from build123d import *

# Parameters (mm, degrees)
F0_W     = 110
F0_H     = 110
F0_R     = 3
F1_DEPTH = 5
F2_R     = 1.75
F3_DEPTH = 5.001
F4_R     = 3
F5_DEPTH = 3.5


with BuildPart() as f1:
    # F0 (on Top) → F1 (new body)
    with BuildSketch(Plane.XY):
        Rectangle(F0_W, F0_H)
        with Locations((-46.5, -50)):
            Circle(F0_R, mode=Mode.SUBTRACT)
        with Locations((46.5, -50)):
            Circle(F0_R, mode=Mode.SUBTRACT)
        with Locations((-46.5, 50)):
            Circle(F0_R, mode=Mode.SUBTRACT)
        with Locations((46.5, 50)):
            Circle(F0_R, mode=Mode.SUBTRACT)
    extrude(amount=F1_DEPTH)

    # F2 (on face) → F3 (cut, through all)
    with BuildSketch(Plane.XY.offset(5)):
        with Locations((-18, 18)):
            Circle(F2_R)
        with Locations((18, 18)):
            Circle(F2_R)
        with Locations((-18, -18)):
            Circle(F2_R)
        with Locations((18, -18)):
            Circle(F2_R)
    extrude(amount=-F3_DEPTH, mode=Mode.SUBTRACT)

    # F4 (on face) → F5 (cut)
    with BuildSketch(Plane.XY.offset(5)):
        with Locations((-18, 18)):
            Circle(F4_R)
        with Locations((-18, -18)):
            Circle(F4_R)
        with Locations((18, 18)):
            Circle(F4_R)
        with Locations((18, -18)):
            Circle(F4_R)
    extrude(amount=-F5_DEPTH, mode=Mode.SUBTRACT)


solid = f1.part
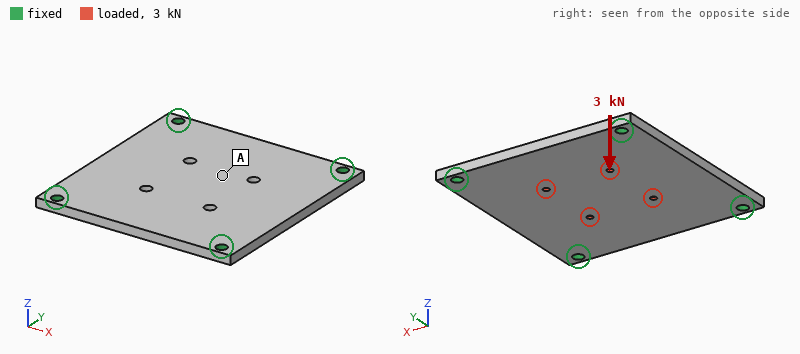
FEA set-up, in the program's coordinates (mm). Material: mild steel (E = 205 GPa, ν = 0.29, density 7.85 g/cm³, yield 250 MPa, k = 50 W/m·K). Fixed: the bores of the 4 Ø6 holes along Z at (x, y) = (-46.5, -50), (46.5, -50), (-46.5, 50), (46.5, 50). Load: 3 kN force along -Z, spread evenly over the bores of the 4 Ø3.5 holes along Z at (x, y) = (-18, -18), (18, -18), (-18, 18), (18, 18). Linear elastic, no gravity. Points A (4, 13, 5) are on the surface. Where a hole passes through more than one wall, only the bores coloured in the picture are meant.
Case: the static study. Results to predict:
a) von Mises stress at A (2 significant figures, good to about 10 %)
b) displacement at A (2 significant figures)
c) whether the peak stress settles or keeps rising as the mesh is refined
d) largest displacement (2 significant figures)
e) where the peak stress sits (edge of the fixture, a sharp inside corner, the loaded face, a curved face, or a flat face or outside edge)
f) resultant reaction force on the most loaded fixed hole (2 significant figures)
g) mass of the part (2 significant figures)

58 MPa
0.12 mm
keeps rising
0.13 mm
edge of the fixture
750 N
470 g
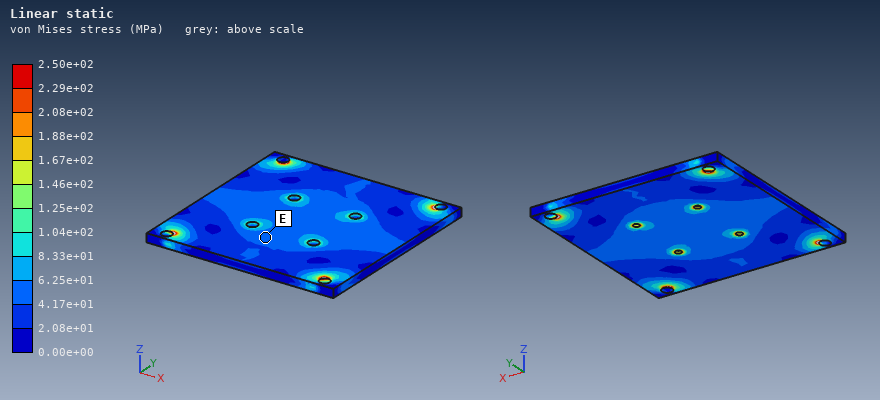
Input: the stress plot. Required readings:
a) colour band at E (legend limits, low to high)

4.17e+01 to 6.25e+01 MPa
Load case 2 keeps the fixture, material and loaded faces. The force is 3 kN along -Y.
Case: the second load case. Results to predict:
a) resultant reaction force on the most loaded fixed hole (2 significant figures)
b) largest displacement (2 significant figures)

830 N
2.9 µm
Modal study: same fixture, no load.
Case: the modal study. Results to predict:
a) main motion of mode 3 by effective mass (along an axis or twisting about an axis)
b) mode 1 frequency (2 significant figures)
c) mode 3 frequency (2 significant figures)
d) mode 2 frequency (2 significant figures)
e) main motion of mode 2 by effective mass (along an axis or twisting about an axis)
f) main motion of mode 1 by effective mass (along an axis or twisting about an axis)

twisting about X
1800 Hz
3300 Hz
3000 Hz
twisting about Y
along Z
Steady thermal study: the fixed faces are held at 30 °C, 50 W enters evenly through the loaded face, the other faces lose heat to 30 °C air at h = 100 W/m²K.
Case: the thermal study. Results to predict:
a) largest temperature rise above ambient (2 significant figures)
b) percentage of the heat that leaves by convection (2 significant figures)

52 K
72 %
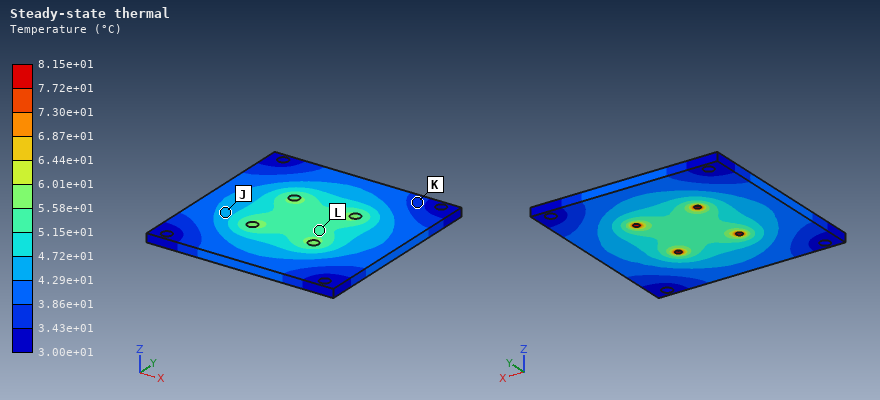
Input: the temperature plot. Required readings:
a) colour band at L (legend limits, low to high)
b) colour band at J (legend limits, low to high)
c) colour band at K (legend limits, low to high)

5.15e+01 to 5.58e+01 °C
4.29e+01 to 4.72e+01 °C
3.43e+01 to 3.86e+01 °C
